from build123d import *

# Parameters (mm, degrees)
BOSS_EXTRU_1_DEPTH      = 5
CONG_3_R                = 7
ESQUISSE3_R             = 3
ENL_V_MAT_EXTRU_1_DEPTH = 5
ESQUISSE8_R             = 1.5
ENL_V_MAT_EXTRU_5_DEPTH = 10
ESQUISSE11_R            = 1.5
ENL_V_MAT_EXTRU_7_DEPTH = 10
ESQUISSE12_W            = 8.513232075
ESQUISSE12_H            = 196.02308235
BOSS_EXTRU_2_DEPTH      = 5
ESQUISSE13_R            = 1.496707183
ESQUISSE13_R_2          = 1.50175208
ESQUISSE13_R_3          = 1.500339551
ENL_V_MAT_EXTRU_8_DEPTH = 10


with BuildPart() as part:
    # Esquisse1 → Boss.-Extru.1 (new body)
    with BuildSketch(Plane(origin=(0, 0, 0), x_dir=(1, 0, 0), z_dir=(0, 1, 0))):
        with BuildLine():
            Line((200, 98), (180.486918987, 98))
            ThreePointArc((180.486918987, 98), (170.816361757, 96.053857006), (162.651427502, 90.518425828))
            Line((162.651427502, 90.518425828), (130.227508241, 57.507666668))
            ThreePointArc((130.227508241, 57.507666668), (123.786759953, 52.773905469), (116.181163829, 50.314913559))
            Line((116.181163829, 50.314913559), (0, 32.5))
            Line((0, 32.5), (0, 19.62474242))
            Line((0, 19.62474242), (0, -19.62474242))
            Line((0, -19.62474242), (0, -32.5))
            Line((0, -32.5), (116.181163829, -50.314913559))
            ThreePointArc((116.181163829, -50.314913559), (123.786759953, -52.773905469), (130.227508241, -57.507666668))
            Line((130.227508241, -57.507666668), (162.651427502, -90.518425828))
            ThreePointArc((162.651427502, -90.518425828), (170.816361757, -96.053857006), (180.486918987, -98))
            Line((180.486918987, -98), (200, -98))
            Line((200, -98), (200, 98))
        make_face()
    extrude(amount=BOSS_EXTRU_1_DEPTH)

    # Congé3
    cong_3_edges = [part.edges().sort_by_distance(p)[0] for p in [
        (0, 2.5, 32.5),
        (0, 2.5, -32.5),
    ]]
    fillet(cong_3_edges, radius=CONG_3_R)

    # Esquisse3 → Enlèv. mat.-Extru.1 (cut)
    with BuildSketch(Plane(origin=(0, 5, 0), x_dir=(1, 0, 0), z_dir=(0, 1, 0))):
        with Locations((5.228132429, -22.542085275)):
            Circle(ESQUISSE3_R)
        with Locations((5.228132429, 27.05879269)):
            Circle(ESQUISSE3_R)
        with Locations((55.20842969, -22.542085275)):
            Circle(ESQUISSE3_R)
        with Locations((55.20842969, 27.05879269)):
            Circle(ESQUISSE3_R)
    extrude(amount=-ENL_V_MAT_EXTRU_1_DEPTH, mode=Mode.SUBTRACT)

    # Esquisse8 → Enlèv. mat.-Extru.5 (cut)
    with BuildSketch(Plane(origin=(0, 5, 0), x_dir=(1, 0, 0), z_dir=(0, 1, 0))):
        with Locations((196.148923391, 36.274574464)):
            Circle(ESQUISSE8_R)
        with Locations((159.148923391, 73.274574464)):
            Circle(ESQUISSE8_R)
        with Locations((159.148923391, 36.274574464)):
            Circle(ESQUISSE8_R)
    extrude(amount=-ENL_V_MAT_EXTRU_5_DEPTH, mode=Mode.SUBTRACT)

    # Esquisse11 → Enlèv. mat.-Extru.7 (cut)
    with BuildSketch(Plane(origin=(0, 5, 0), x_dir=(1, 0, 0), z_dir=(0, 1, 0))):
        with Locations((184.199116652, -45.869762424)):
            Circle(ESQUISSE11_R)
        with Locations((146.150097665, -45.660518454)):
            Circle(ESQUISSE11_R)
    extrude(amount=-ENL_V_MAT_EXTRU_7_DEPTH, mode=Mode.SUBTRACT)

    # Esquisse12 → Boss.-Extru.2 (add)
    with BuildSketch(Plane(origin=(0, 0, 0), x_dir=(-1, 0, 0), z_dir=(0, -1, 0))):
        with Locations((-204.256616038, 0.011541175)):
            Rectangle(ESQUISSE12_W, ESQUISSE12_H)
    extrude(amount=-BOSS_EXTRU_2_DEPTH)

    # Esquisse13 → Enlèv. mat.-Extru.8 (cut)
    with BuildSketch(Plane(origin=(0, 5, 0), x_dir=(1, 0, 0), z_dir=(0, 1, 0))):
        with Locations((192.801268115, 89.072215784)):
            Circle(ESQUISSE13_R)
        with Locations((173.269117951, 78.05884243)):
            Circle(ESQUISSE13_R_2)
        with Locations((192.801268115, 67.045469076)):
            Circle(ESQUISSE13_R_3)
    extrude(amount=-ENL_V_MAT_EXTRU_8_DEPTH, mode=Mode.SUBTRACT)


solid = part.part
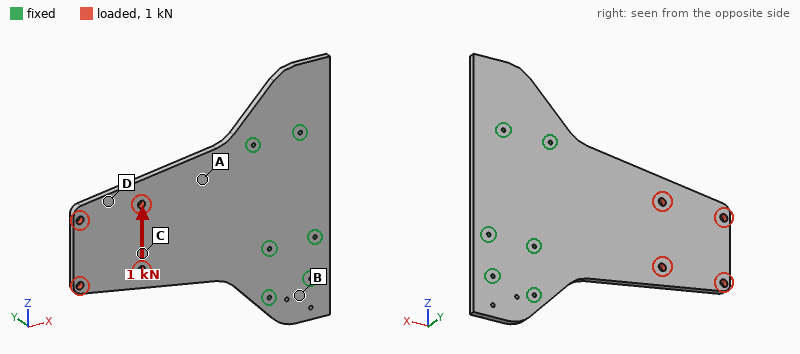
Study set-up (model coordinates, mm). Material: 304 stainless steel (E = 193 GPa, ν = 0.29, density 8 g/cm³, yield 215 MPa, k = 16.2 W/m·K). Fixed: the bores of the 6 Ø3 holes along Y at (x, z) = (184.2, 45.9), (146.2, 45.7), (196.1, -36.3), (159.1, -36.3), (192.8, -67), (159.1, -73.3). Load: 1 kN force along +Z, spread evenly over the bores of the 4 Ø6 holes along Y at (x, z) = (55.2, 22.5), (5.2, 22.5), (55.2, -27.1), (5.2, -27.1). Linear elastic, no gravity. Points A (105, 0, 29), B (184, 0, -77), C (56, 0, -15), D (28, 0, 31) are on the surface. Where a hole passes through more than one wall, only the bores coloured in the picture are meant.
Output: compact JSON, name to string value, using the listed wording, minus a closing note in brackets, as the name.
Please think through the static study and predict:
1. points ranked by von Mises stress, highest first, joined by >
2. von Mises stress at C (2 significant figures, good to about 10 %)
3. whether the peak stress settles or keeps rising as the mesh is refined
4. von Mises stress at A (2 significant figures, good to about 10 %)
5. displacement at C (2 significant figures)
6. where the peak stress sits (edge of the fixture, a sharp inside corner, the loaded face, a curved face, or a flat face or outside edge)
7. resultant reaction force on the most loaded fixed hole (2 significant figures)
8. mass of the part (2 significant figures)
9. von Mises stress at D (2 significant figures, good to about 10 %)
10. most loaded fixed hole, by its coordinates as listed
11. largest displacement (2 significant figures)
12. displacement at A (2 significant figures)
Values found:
{"points ranked by von Mises stress, highest first, joined by >": "A > C > D > B", "von Mises stress at C": "4.9 MPa", "whether the peak stress settles or keeps rising as the mesh is refined": "keeps rising", "von Mises stress at A": "6.3 MPa", "displacement at C": "7.3 µm", "where the peak stress sits": "edge of the fixture", "resultant reaction force on the most loaded fixed hole": "1.1 kN", "mass of the part": "990 g", "von Mises stress at D": "2.8 MPa", "most loaded fixed hole, by its coordinates as listed": "(146.2, 45.7)", "largest displacement": "15 µm", "displacement at A": "2.6 µm"}
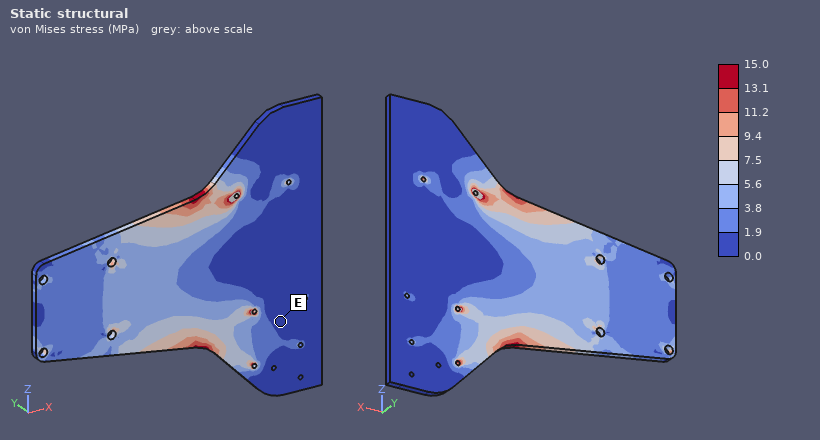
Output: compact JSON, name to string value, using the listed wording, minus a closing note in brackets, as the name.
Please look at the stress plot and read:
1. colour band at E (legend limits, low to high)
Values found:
{"colour band at E": "0.0 to 1.9 MPa"}
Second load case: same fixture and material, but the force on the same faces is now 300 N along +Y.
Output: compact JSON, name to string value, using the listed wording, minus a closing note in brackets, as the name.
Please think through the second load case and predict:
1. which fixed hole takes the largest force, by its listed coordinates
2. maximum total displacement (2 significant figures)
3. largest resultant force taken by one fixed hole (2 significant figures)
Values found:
{"which fixed hole takes the largest force, by its listed coordinates": "(146.2, 45.7)", "maximum total displacement": "1.3 mm", "largest resultant force taken by one fixed hole": "470 N"}
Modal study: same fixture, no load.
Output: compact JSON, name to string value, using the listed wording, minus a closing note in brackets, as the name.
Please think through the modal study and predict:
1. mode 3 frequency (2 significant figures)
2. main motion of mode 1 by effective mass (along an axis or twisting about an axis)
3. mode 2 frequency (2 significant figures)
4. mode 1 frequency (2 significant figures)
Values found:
{"mode 3 frequency": "1100 Hz", "main motion of mode 1 by effective mass": "along Y", "mode 2 frequency": "850 Hz", "mode 1 frequency": "200 Hz"}
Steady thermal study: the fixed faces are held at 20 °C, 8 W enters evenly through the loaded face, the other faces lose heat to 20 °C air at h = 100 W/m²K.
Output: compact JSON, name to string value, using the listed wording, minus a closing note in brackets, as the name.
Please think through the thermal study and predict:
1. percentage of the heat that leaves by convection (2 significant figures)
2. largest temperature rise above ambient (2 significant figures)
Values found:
{"percentage of the heat that leaves by convection": "100 %", "largest temperature rise above ambient": "22 K"}
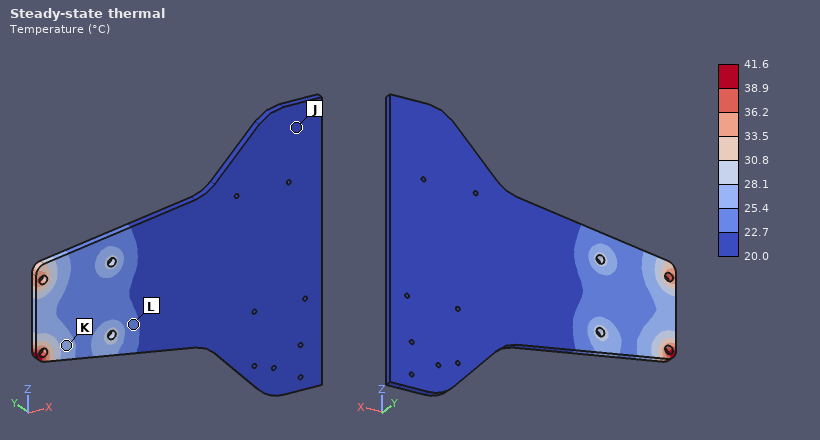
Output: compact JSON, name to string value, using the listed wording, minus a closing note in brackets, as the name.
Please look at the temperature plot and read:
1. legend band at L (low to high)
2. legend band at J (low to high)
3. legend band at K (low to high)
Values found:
{"legend band at L": "22.7 to 25.4 °C", "legend band at J": "20.0 to 22.7 °C", "legend band at K": "25.4 to 28.1 °C"}
